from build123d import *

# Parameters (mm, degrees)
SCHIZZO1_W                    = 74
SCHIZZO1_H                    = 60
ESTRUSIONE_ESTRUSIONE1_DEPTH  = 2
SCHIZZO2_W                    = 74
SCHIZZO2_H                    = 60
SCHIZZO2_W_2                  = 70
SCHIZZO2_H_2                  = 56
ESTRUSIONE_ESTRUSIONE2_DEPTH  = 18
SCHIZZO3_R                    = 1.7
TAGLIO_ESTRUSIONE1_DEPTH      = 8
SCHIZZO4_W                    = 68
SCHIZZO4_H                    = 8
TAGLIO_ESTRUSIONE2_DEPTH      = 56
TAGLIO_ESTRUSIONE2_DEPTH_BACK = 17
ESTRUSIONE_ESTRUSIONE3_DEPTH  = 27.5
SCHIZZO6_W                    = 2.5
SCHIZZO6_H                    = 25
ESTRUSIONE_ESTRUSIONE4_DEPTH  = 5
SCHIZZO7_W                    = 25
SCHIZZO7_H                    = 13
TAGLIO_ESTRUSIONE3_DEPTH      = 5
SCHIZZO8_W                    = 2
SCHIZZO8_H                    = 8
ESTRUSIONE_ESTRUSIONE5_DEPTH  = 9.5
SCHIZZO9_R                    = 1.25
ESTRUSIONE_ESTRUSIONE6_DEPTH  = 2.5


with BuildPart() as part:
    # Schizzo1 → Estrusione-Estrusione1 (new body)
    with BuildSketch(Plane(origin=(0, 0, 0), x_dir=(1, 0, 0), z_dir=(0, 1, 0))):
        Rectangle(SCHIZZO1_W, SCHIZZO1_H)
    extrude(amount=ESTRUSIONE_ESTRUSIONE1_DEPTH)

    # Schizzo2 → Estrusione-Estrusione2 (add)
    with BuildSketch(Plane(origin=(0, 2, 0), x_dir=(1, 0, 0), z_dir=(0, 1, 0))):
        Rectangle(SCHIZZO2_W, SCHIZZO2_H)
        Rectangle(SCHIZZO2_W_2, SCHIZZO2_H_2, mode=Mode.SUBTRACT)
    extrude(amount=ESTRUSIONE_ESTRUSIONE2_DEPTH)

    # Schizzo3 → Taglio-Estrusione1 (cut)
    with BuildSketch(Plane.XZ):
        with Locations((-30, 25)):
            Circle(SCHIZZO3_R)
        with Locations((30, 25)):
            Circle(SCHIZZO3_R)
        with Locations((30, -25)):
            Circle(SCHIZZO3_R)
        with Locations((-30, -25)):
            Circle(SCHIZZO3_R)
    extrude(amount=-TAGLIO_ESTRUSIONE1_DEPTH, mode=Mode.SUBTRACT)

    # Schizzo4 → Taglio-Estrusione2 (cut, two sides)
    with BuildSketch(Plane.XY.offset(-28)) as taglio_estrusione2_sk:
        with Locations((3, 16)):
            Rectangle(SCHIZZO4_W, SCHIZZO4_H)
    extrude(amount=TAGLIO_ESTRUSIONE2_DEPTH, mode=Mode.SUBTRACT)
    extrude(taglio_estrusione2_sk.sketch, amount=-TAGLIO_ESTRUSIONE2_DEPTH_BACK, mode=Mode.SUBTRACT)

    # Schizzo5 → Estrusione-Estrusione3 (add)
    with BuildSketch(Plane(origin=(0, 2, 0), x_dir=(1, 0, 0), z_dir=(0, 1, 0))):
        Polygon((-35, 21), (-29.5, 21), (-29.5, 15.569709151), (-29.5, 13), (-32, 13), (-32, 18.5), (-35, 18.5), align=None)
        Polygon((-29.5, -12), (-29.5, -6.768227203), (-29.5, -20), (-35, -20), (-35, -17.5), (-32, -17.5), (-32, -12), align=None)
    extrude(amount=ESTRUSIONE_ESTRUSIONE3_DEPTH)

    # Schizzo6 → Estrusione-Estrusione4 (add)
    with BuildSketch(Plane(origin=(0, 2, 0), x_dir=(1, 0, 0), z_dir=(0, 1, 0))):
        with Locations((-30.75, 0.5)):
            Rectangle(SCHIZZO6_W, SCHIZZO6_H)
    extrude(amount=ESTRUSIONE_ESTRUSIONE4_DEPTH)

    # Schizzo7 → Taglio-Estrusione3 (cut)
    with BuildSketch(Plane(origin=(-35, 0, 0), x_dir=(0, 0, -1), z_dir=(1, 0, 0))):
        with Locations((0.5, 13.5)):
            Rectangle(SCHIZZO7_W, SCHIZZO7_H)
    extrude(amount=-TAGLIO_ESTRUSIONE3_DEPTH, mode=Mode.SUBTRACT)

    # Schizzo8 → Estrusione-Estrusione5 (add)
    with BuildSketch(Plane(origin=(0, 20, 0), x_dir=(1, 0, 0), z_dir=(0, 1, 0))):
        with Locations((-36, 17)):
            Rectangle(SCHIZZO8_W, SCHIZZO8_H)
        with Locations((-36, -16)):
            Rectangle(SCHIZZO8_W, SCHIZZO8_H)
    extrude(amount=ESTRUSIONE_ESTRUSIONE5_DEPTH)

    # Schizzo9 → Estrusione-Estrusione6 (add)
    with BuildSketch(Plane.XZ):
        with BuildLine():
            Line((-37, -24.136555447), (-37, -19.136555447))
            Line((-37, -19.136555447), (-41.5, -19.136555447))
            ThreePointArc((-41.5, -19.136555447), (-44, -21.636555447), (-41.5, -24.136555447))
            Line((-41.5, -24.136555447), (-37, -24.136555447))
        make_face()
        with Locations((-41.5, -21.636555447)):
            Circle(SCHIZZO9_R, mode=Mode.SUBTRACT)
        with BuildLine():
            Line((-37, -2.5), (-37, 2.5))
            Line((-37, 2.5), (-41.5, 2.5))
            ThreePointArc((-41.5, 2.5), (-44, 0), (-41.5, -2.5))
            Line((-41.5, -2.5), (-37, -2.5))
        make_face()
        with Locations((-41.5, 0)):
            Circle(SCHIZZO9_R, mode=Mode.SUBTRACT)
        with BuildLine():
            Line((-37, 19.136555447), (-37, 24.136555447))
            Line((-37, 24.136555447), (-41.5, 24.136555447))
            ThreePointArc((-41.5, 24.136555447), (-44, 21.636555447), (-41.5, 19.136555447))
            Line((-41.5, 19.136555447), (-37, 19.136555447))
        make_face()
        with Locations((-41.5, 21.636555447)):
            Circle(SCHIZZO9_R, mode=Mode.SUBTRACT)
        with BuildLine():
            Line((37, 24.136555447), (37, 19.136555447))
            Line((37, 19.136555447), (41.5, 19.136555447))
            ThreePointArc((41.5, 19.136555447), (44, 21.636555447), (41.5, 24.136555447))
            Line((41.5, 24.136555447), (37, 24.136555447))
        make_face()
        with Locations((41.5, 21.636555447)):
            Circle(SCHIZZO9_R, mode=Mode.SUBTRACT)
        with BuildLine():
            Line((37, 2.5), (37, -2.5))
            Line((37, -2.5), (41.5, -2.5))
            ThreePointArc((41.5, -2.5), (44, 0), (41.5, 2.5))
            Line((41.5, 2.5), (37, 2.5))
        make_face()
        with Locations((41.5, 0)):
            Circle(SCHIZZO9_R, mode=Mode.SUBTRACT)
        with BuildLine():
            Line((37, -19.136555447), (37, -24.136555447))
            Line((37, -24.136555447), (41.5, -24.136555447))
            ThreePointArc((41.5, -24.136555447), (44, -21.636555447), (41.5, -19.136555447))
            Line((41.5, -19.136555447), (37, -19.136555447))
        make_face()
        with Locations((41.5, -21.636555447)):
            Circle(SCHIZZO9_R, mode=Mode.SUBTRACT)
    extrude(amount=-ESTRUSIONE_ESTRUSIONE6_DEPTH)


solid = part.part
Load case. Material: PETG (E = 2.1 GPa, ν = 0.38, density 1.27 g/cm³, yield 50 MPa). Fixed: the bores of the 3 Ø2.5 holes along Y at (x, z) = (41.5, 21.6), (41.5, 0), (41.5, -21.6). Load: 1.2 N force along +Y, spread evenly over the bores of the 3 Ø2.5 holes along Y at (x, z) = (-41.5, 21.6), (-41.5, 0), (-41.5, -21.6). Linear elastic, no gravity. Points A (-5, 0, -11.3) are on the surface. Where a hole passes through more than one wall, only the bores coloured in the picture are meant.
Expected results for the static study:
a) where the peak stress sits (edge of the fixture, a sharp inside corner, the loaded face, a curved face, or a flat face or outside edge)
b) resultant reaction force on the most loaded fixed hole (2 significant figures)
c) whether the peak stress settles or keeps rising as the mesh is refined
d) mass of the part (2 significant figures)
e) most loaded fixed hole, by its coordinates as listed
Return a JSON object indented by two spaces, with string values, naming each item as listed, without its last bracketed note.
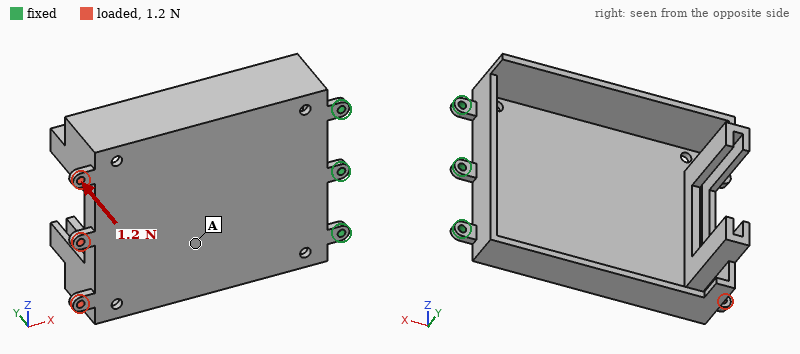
{
  "where the peak stress sits": "edge of the fixture",
  "resultant reaction force on the most loaded fixed hole": "2.7 N",
  "whether the peak stress settles or keeps rising as the mesh is refined": "keeps rising",
  "mass of the part": "23 g",
  "most loaded fixed hole, by its coordinates as listed": "(41.5, 0)"
}
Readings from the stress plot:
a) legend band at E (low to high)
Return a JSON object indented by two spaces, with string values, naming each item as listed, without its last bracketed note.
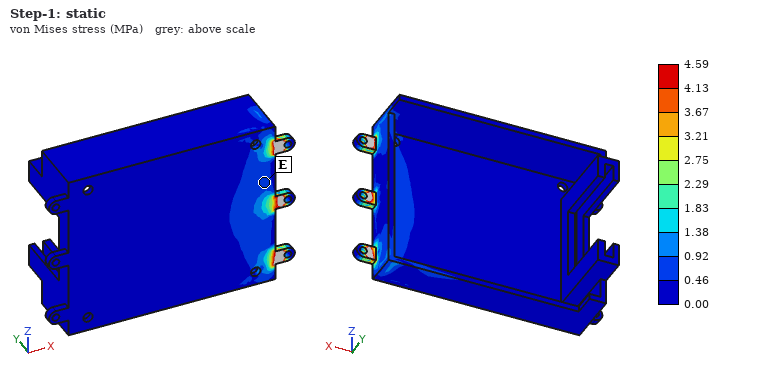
{
  "legend band at E": "0.46 to 0.92 MPa"
}
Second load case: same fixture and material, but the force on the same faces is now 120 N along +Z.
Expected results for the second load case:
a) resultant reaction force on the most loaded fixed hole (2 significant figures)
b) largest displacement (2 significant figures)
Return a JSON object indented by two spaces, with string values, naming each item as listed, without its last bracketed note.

{
  "resultant reaction force on the most loaded fixed hole": "220 N",
  "largest displacement": "0.94 mm"
}
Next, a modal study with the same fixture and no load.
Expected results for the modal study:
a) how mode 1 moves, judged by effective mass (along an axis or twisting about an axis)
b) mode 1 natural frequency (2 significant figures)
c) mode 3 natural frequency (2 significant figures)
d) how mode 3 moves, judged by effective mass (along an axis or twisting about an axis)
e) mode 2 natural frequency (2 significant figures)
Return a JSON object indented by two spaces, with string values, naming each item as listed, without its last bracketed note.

{
  "how mode 1 moves, judged by effective mass": "along Y",
  "mode 1 natural frequency": "54 Hz",
  "mode 3 natural frequency": "700 Hz",
  "how mode 3 moves, judged by effective mass": "along Z",
  "mode 2 natural frequency": "150 Hz"
}
